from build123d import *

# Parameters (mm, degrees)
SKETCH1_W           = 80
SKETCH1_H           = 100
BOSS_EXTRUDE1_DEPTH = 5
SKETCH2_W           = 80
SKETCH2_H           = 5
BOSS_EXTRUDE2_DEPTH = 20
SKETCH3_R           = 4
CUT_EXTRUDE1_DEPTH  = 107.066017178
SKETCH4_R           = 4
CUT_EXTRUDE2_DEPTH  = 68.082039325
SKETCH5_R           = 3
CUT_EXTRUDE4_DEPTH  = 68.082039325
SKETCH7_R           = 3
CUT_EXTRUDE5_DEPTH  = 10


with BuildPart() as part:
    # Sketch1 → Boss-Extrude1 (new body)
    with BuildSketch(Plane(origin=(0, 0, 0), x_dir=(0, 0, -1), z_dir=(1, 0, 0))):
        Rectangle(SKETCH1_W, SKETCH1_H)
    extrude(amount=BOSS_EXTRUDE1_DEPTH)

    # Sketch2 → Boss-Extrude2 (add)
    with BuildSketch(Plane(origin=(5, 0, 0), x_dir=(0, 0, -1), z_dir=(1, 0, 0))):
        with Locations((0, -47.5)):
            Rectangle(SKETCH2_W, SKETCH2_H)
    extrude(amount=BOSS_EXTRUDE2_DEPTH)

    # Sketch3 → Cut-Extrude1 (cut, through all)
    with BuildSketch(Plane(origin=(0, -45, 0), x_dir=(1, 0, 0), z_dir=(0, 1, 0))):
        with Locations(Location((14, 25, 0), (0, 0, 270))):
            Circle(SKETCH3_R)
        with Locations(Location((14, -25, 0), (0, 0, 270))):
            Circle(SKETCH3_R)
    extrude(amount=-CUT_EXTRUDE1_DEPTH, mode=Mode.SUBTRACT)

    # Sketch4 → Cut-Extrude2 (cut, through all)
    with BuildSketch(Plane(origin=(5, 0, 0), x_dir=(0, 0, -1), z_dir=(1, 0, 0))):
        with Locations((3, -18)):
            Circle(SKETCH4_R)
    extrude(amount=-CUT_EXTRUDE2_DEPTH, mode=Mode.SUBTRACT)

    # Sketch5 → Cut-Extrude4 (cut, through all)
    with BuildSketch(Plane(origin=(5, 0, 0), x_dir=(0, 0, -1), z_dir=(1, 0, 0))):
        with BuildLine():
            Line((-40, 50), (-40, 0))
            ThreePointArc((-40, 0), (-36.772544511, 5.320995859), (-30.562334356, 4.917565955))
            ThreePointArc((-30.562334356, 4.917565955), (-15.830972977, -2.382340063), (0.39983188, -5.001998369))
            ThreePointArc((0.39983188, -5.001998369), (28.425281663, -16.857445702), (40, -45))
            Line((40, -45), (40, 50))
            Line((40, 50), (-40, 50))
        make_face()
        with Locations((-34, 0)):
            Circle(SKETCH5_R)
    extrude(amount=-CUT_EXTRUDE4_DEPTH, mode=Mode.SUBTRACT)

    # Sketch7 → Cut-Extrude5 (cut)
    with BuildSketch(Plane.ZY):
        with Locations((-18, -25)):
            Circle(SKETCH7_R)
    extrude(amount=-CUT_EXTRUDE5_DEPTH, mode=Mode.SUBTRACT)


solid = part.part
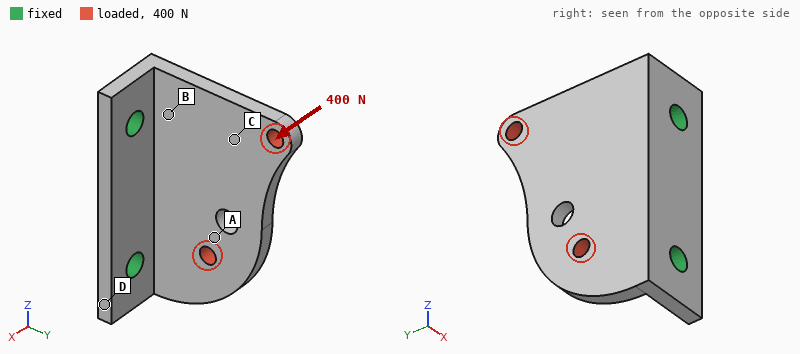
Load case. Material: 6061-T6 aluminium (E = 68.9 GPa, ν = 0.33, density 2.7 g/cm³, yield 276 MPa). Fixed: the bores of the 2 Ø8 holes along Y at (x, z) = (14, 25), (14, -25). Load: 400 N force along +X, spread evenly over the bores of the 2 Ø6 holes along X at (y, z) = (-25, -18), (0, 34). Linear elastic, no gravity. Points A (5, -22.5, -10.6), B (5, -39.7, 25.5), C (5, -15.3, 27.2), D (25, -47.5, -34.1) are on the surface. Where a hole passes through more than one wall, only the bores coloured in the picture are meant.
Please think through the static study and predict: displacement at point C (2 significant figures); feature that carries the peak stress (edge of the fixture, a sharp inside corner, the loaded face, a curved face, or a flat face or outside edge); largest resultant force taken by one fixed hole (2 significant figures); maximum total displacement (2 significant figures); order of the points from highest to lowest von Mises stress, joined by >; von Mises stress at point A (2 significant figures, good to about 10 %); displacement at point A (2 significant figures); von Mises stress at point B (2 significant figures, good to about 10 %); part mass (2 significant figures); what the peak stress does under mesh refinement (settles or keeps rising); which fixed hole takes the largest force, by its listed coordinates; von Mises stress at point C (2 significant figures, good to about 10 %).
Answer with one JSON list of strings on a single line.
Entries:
["0.20 mm", "edge of the fixture", "250 N", "0.42 mm", "B > C > A > D", "13 MPa", "0.099 mm", "36 MPa", "65 g", "keeps rising", "(14, 25)", "26 MPa"]
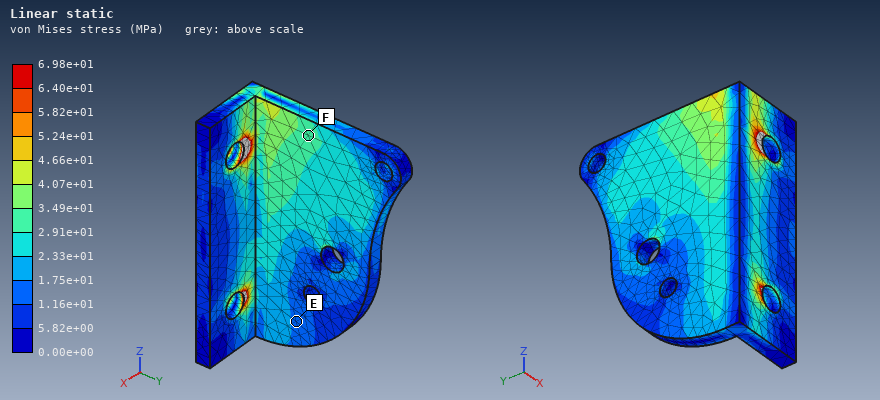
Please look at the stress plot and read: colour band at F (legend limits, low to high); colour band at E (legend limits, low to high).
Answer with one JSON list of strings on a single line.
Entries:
["2.91e+01 to 3.49e+01 MPa", "1.16e+01 to 1.75e+01 MPa"]
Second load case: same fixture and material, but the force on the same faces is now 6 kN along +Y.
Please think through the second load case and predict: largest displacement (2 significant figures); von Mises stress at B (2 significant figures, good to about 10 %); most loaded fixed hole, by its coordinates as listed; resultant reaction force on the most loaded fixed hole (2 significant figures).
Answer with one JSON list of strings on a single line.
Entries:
["0.40 mm", "54 MPa", "(14, 25)", "3.9 kN"]
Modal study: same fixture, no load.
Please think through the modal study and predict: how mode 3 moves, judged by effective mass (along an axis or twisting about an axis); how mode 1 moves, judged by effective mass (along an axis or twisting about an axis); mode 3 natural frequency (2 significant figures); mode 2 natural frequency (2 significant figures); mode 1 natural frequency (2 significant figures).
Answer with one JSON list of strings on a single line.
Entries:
["along Z", "along X", "6500 Hz", "3500 Hz", "1600 Hz"]
